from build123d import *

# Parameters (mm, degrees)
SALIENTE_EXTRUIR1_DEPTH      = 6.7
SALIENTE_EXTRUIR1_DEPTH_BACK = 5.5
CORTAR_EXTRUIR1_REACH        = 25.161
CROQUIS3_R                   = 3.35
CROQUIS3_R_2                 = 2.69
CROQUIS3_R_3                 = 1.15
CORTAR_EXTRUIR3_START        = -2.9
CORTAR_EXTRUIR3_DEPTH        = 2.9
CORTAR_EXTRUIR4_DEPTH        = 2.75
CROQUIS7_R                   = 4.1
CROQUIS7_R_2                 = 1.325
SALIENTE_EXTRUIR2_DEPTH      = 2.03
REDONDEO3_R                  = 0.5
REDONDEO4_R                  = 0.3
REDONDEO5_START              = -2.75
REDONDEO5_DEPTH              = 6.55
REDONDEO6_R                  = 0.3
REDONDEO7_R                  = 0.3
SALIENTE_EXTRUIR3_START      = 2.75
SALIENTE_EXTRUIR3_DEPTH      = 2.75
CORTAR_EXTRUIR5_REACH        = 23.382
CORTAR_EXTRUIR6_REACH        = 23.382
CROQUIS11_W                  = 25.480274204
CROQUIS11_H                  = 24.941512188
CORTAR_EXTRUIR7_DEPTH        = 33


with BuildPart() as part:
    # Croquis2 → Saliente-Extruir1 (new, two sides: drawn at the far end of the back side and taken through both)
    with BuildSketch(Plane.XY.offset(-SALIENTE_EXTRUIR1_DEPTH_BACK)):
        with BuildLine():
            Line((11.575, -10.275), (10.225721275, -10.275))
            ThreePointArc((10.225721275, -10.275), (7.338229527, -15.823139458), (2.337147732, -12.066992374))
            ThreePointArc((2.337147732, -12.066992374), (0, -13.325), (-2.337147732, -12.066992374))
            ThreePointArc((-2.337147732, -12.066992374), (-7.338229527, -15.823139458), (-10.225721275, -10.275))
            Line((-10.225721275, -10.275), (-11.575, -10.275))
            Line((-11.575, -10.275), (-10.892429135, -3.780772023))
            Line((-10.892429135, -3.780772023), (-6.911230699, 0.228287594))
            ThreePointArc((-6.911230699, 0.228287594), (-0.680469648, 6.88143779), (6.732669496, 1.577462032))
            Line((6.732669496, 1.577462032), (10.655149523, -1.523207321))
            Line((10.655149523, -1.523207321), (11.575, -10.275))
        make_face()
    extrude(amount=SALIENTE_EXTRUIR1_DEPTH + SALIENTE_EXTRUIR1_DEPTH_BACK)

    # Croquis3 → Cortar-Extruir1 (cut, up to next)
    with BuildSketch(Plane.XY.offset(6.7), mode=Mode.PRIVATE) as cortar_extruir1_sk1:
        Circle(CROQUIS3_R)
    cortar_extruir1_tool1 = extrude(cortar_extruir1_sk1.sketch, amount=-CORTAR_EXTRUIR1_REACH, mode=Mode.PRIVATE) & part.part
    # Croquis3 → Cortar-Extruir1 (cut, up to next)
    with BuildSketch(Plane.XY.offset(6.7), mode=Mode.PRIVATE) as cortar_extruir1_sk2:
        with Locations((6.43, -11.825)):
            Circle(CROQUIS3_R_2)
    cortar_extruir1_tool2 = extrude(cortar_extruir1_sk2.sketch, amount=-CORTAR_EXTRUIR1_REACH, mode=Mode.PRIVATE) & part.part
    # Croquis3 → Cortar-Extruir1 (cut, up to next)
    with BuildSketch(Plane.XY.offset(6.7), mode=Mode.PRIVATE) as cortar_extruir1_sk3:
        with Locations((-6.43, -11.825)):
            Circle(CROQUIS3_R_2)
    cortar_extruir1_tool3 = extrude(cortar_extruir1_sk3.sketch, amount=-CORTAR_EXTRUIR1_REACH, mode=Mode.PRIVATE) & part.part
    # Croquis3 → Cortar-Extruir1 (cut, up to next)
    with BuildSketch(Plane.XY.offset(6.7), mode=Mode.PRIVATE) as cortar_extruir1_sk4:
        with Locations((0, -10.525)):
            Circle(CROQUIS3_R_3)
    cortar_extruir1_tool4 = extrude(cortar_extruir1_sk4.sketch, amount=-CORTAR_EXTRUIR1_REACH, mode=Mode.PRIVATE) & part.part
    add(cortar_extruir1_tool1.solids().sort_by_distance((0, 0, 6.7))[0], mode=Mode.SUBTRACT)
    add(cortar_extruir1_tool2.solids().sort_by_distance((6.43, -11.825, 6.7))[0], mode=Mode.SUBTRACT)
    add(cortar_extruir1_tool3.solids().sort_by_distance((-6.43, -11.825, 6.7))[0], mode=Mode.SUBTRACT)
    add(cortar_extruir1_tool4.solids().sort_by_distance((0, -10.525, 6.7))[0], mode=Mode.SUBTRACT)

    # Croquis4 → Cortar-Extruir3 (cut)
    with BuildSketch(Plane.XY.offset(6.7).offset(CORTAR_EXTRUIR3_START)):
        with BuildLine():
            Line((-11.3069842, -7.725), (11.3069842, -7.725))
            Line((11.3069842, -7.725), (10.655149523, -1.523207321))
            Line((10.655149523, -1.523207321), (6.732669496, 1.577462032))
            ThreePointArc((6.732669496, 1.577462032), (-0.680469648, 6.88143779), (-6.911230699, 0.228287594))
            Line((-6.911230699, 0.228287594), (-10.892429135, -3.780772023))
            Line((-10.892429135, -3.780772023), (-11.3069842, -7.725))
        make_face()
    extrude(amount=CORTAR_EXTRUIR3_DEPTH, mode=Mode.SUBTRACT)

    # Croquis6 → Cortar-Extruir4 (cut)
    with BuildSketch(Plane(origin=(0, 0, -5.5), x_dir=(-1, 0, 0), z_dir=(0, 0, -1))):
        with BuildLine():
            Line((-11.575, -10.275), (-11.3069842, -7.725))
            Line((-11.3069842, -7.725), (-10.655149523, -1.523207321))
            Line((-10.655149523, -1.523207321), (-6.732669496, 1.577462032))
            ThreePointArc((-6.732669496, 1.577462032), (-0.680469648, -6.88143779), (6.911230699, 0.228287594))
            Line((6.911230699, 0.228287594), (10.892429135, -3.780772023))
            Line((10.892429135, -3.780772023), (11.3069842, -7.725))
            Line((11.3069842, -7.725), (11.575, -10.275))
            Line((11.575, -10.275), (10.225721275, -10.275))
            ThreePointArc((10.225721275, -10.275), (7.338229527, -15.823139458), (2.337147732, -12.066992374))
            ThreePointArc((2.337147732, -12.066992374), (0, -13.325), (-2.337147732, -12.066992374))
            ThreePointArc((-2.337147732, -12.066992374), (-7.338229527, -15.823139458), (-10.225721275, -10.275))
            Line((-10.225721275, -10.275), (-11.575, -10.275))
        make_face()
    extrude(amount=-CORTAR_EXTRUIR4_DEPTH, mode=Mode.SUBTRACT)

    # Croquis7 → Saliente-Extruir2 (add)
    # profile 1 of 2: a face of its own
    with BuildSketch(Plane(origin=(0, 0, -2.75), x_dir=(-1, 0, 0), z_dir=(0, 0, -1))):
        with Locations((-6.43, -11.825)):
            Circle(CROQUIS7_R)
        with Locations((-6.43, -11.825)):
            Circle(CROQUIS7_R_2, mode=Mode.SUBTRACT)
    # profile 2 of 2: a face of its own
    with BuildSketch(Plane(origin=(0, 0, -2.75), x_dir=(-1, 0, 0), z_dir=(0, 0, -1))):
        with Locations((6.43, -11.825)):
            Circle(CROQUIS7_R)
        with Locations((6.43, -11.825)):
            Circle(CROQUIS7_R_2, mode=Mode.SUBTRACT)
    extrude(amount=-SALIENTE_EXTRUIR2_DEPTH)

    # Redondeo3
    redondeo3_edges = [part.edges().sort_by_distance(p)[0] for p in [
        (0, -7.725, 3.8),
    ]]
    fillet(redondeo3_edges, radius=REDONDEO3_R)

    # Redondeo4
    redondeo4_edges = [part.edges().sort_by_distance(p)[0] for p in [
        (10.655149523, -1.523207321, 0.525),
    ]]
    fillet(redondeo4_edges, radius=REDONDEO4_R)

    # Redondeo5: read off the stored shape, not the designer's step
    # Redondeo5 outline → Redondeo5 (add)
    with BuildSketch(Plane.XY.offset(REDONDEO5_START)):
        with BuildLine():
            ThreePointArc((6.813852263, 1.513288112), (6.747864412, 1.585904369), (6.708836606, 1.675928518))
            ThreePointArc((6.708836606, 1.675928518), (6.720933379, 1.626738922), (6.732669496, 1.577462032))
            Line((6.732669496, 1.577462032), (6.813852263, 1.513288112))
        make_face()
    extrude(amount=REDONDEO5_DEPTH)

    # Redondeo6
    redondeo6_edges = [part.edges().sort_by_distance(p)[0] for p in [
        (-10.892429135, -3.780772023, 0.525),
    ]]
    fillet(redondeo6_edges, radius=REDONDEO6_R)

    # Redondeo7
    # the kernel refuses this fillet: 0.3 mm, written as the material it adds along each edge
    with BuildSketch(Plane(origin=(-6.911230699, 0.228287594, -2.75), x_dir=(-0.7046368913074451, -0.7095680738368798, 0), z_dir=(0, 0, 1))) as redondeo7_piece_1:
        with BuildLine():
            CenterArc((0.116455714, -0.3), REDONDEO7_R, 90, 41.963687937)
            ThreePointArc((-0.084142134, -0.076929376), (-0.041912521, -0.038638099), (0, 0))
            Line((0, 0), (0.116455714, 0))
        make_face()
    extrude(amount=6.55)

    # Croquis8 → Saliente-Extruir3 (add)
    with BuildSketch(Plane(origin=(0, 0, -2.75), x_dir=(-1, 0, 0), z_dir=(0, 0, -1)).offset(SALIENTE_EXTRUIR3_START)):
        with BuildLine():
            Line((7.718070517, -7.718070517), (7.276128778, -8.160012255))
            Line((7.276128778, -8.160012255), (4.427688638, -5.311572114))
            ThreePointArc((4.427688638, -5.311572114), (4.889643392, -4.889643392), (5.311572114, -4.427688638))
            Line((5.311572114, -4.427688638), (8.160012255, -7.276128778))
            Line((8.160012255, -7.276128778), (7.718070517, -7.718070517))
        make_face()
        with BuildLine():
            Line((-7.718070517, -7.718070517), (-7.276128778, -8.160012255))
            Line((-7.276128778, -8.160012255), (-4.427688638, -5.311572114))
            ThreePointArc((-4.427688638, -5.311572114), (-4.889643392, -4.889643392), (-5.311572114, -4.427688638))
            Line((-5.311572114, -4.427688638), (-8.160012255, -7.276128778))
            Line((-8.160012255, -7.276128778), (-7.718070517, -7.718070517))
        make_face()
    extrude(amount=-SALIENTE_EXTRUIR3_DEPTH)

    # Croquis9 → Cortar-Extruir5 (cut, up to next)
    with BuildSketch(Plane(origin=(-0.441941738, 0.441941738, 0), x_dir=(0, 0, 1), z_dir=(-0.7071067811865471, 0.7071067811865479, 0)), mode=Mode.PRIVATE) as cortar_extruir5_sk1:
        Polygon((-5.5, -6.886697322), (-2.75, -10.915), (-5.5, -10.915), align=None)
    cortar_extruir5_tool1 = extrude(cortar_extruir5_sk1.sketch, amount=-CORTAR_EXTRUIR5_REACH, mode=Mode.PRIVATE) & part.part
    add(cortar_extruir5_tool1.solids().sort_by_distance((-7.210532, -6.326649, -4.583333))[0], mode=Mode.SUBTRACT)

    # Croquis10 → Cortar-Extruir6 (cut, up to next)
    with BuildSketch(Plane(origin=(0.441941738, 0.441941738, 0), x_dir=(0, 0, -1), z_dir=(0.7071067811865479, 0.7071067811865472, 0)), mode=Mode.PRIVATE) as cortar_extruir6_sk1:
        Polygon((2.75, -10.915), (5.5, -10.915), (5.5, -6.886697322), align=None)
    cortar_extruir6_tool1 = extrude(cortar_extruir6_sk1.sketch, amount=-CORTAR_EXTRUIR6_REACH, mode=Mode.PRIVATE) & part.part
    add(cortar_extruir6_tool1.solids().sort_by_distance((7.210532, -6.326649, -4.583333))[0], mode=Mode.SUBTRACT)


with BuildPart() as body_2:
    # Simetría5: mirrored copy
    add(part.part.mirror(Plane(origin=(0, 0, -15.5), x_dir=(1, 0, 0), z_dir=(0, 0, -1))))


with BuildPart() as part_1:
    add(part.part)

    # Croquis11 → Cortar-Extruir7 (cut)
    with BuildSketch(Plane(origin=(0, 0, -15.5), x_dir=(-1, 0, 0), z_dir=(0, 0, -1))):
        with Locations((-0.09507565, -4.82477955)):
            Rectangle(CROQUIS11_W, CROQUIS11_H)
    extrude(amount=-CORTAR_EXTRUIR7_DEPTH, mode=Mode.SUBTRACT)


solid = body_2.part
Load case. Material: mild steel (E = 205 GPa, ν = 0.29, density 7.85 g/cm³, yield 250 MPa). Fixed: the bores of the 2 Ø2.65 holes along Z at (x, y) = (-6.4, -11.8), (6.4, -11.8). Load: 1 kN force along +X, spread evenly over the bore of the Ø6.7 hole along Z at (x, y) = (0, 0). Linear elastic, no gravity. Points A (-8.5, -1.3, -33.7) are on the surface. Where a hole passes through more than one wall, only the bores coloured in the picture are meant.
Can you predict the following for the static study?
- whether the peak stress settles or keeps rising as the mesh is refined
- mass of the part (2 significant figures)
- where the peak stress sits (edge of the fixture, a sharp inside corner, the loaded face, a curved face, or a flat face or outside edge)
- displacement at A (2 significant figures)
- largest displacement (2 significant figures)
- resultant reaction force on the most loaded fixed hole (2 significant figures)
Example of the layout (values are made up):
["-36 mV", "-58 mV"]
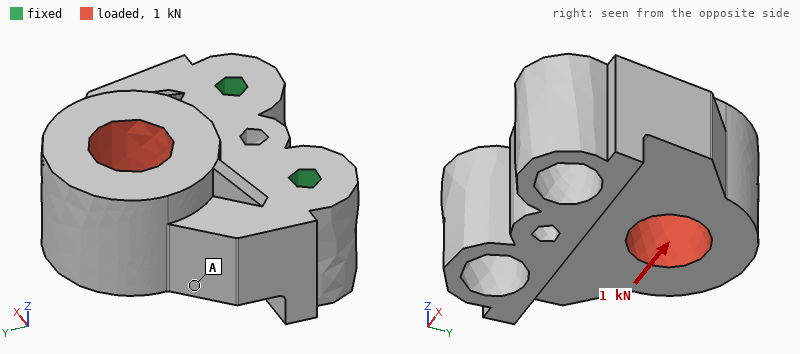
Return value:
["keeps rising", "21 g", "edge of the fixture", "3.8 µm", "6.3 µm", "940 N"]
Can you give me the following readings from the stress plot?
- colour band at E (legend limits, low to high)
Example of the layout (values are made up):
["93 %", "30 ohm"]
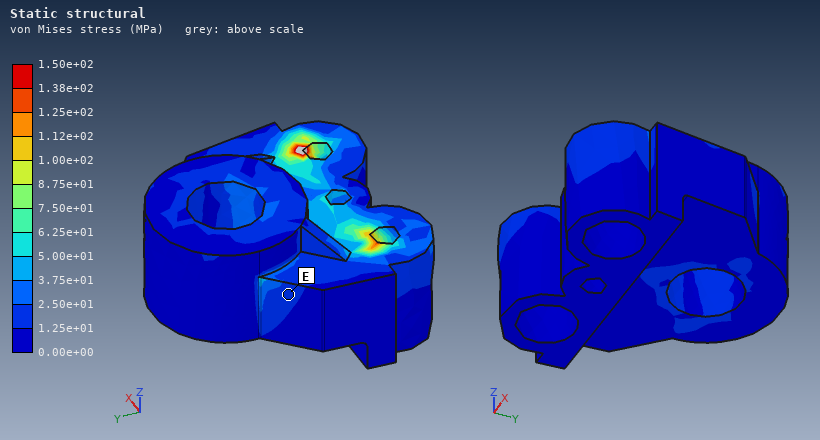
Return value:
["1.25e+01 to 2.50e+01 MPa"]
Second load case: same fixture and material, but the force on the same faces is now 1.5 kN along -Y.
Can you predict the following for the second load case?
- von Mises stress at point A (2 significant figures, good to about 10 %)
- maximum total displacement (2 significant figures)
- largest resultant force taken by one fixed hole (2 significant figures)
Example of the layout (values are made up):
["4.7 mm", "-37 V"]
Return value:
["7.2 MPa", "5.5 µm", "770 N"]
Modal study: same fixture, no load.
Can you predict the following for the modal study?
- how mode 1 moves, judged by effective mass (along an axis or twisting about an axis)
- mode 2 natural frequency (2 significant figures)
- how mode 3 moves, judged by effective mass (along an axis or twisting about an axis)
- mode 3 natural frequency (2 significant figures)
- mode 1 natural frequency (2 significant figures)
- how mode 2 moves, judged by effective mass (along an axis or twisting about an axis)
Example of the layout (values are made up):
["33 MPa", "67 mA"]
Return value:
["along Z", "22 kHz", "along X", "27 kHz", "7200 Hz", "along X"]
